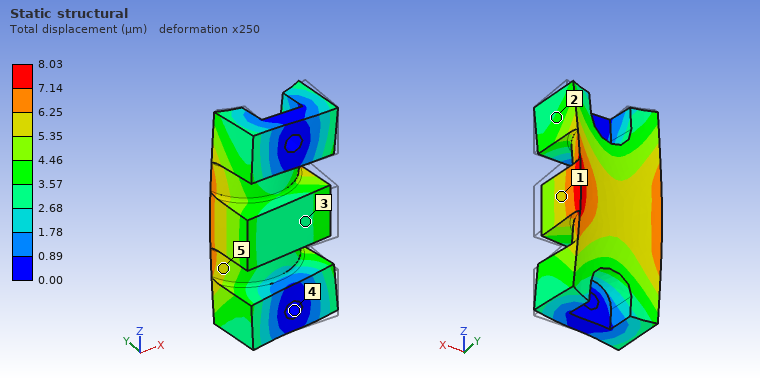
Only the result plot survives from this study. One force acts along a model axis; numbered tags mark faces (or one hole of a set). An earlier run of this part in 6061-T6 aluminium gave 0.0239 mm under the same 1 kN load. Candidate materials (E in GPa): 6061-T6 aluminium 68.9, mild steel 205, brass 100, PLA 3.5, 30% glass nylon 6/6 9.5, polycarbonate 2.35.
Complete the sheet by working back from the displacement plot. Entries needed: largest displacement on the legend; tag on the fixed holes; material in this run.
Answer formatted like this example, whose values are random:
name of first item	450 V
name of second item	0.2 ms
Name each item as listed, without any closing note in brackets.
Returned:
largest displacement on the legend	8.03 µm
tag on the fixed holes	4
material in this run	mild steel
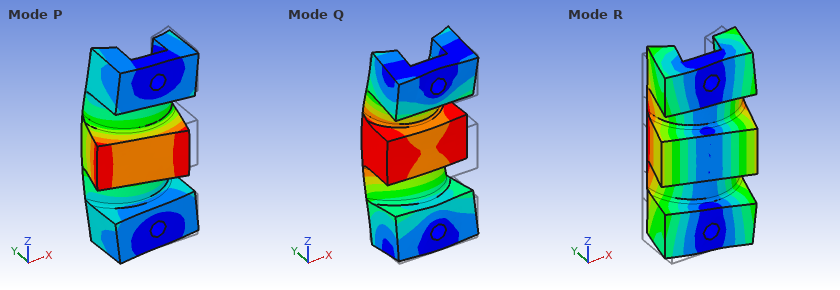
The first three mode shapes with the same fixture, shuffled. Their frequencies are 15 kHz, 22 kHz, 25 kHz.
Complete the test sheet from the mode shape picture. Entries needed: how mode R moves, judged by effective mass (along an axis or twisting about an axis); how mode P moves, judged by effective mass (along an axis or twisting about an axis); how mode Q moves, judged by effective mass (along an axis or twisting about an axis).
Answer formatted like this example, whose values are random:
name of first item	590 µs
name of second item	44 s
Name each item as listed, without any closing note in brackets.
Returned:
how mode R moves, judged by effective mass	along X
how mode P moves, judged by effective mass	along X
how mode Q moves, judged by effective mass	along Y
